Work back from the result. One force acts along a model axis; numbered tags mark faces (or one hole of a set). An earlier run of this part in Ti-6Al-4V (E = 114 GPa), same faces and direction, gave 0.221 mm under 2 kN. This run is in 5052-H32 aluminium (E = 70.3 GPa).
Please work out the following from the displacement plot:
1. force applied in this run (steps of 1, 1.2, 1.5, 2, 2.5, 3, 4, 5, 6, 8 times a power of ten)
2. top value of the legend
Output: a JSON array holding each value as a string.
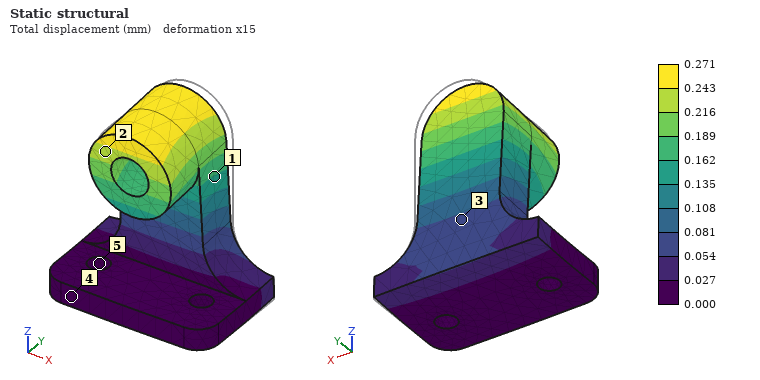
["1.5 kN", "0.271 mm"]
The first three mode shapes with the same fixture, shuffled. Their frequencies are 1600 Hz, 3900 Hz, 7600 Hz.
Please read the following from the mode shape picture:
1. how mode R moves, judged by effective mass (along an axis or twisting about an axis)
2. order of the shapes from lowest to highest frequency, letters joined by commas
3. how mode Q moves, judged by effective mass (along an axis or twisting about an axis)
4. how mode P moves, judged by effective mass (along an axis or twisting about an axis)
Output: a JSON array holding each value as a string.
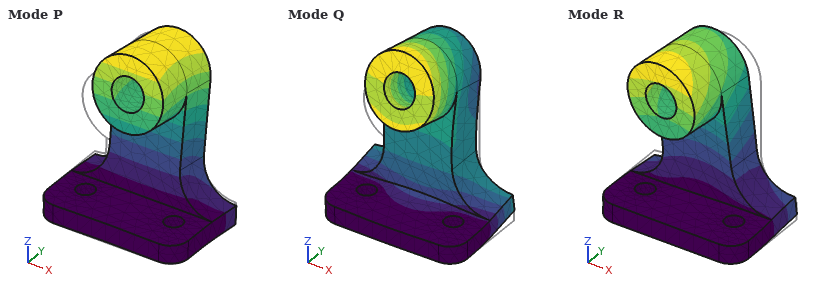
["along X", "P, R, Q", "along Z", "along Y"]
